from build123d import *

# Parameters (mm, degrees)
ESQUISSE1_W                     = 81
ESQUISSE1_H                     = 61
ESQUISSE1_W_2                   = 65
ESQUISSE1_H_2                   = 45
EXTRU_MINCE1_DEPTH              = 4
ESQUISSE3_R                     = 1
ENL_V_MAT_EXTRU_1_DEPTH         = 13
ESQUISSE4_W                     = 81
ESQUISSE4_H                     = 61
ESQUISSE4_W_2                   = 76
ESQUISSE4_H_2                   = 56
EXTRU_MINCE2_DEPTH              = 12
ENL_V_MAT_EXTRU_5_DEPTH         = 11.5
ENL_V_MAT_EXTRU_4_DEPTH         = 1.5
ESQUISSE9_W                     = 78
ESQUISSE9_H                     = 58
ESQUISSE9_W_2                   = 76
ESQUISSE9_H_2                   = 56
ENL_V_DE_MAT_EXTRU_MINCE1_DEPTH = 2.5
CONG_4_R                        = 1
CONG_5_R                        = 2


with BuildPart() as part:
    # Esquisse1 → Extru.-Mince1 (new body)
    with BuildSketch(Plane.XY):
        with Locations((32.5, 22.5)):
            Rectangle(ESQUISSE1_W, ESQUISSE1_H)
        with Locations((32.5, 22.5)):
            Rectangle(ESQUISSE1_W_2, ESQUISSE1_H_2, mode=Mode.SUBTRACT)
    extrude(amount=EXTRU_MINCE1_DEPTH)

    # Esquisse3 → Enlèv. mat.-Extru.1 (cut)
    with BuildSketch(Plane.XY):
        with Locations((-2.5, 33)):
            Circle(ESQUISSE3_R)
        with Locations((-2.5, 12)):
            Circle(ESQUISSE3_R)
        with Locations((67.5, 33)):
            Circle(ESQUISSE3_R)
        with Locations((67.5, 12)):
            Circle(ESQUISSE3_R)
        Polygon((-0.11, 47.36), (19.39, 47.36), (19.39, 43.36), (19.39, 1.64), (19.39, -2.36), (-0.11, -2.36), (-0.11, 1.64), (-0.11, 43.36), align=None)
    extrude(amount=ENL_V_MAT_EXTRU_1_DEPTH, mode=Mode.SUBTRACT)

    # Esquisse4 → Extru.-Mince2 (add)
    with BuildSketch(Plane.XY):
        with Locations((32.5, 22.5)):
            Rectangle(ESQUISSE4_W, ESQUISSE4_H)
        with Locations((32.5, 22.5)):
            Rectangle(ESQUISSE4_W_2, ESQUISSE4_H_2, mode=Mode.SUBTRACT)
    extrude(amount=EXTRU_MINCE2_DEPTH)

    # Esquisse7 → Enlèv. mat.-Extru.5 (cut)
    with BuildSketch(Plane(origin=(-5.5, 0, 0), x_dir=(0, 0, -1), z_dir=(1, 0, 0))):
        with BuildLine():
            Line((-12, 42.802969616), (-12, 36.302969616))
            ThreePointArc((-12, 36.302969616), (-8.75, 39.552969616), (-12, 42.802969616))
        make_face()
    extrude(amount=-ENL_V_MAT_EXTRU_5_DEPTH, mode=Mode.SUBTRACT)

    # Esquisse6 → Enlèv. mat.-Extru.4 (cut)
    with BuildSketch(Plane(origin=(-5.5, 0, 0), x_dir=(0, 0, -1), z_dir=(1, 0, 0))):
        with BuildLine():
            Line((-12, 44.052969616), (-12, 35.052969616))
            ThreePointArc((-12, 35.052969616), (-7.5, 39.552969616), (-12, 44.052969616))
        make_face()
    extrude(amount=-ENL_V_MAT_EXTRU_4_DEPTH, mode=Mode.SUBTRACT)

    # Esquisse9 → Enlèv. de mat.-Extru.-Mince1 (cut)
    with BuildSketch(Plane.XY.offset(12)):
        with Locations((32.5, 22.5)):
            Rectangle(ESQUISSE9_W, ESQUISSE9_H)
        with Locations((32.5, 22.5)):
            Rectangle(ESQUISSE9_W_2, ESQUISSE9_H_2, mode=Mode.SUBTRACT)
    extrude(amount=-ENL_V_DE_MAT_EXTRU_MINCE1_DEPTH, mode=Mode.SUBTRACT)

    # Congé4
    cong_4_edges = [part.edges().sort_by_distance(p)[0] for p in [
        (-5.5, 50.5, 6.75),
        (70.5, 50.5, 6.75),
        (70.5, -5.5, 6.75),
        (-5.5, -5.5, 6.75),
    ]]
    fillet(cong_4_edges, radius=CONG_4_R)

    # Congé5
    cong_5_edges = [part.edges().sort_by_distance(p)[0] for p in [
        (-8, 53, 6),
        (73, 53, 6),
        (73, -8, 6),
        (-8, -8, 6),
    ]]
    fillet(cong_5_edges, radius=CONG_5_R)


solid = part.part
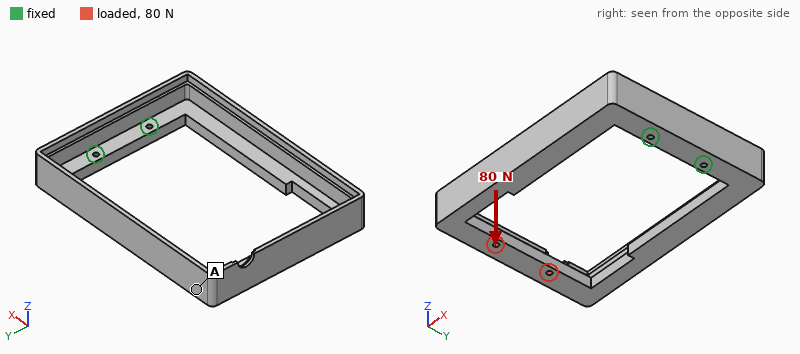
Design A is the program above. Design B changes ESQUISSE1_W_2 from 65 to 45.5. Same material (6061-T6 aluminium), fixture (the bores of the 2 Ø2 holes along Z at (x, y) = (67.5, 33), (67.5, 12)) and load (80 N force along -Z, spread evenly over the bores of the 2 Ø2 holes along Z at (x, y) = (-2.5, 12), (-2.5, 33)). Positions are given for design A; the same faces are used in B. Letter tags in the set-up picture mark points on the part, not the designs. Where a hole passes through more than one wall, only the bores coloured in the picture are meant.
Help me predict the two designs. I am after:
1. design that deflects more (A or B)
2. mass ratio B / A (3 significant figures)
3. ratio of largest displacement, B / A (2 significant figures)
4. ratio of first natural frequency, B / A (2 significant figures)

A
1.14
0.50
1.4
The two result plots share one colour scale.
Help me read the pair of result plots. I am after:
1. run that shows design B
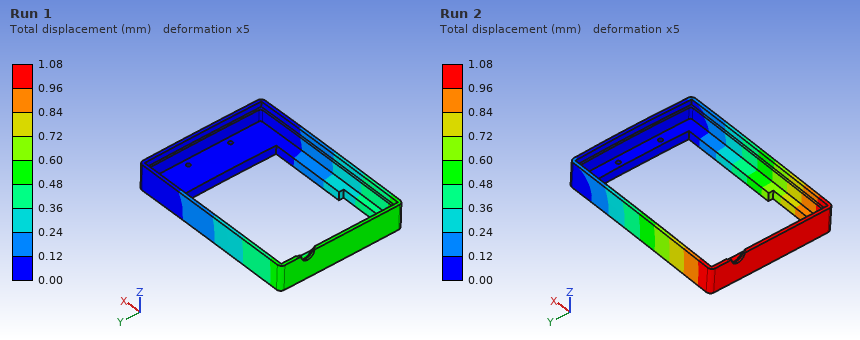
Run 1
